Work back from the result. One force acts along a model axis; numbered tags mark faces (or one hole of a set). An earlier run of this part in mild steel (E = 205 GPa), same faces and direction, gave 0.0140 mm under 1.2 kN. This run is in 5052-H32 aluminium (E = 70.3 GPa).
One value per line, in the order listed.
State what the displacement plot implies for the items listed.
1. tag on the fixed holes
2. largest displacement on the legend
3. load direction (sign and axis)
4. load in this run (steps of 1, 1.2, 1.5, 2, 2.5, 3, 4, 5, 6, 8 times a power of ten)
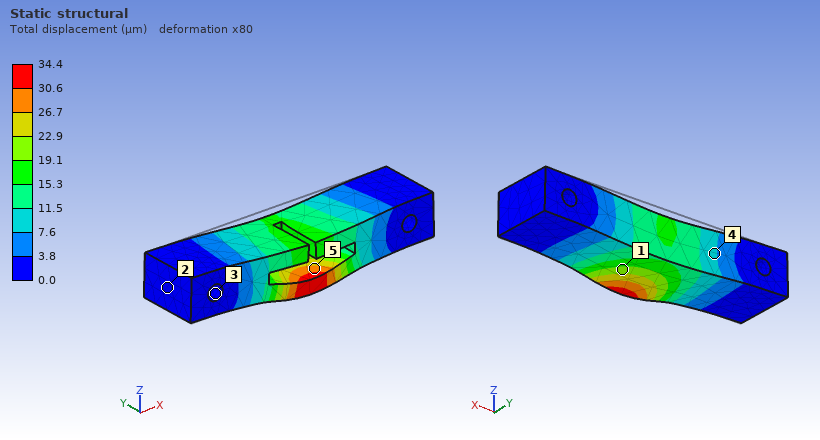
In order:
3
34.4 µm
-Z
1 kN
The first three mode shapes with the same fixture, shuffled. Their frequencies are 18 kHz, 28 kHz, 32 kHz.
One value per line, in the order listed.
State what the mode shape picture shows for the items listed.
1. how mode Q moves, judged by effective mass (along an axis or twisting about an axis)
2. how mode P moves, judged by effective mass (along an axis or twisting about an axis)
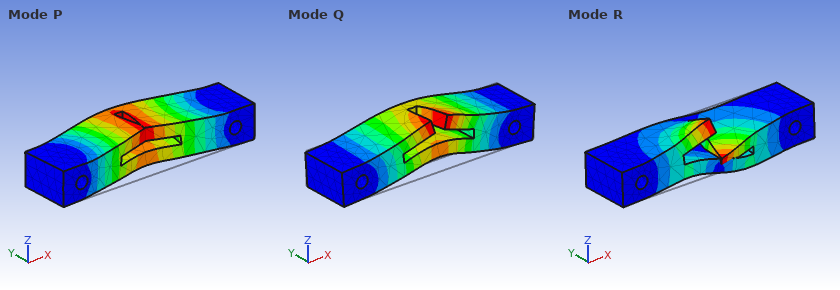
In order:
along Z
along Y
